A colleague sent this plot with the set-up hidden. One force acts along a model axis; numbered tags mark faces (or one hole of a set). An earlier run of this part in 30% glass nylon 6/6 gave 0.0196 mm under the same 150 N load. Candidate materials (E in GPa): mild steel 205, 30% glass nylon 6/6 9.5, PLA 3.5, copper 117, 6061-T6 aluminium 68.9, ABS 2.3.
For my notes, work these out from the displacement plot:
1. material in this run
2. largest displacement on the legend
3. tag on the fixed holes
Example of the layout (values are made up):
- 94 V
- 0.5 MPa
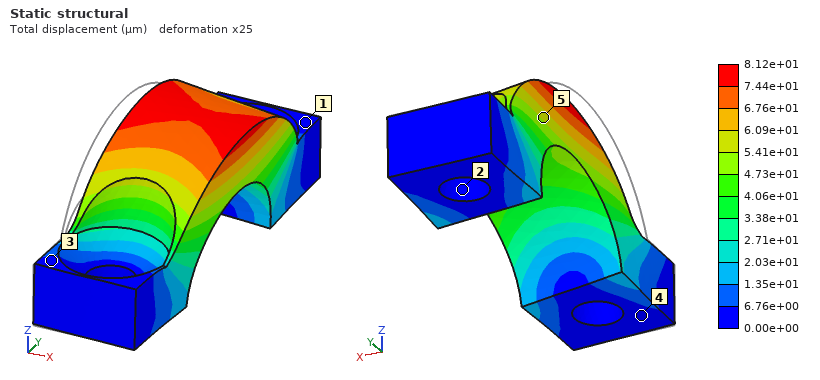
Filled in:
- ABS
- 8.12e+01 µm
- 2
